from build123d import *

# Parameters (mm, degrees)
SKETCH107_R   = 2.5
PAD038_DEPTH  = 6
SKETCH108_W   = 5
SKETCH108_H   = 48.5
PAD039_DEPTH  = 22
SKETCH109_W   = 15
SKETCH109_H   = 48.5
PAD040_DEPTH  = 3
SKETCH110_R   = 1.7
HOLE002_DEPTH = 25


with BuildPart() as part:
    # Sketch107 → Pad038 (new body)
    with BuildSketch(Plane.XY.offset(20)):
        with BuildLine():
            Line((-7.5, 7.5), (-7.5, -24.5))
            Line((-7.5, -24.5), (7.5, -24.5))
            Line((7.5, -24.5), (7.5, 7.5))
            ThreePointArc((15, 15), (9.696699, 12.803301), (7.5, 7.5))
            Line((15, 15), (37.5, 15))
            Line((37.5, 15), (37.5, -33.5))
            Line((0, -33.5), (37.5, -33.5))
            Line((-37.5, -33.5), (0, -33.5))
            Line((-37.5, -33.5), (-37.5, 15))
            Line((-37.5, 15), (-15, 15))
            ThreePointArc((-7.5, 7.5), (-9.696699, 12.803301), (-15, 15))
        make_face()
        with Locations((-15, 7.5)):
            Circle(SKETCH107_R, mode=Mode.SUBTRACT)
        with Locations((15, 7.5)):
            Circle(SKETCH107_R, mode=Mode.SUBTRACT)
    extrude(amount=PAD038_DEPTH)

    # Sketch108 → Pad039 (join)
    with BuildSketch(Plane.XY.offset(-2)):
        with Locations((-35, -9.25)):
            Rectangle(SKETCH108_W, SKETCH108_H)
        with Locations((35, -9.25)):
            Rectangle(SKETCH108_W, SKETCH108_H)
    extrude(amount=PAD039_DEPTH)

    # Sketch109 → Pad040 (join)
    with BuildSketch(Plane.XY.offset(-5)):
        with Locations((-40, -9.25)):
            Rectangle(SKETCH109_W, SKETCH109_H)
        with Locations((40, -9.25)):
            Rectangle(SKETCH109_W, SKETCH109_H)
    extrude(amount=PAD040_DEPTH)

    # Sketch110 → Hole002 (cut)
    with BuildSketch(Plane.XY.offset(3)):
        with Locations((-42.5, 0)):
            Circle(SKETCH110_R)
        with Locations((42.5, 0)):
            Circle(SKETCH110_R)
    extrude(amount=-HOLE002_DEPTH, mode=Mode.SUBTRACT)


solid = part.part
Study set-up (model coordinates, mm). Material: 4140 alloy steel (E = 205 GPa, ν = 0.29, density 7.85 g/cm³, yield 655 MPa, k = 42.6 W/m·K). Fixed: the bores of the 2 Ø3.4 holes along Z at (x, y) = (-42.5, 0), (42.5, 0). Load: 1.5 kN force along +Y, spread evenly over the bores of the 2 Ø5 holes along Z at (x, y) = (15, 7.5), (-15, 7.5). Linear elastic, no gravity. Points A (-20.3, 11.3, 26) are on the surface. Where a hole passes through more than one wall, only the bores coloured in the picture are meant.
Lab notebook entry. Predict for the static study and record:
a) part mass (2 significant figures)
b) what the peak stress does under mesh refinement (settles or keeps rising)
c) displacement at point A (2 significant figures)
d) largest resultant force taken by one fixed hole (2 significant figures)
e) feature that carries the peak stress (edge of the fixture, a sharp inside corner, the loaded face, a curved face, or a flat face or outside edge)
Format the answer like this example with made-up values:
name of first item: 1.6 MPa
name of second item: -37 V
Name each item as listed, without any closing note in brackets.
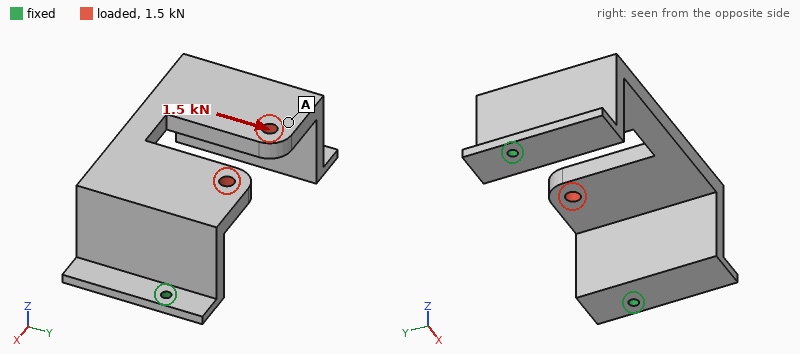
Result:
part mass: 260 g
what the peak stress does under mesh refinement: keeps rising
displacement at point A: 0.23 mm
largest resultant force taken by one fixed hole: 760 N
feature that carries the peak stress: edge of the fixture
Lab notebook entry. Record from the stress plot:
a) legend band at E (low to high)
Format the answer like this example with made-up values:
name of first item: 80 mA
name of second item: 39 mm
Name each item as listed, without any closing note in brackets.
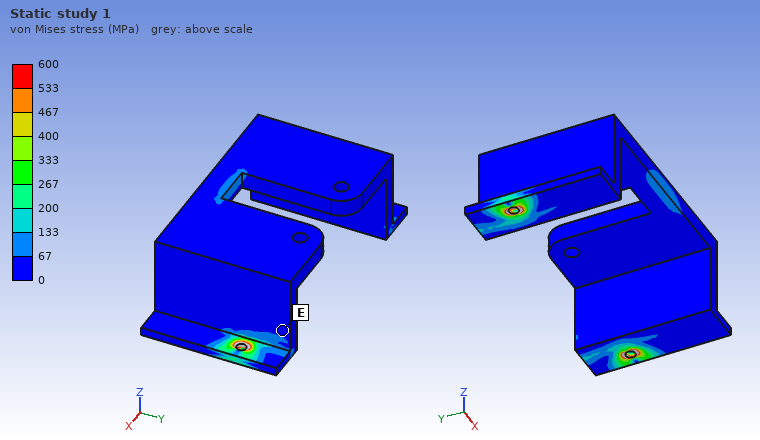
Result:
legend band at E: 0 to 67 MPa
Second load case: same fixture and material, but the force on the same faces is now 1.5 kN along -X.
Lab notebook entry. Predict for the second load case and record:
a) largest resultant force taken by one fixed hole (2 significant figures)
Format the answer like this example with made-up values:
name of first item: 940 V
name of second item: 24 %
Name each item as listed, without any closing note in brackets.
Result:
largest resultant force taken by one fixed hole: 830 N
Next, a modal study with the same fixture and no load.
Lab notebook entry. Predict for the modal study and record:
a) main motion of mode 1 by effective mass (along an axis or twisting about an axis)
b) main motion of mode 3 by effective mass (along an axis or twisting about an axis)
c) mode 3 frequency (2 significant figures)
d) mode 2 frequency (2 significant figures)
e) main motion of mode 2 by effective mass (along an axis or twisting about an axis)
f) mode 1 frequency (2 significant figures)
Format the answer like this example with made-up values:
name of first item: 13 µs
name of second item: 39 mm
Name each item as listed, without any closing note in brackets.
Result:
main motion of mode 1 by effective mass: along Y
main motion of mode 3 by effective mass: along X
mode 3 frequency: 2000 Hz
mode 2 frequency: 1500 Hz
main motion of mode 2 by effective mass: along X
mode 1 frequency: 860 Hz
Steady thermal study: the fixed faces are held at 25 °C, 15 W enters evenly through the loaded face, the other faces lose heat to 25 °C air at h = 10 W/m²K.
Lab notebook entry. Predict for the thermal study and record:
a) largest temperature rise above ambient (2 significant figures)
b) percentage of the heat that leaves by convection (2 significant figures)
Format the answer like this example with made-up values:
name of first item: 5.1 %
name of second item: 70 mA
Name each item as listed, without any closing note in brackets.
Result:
largest temperature rise above ambient: 57 K
percentage of the heat that leaves by convection: 29 %
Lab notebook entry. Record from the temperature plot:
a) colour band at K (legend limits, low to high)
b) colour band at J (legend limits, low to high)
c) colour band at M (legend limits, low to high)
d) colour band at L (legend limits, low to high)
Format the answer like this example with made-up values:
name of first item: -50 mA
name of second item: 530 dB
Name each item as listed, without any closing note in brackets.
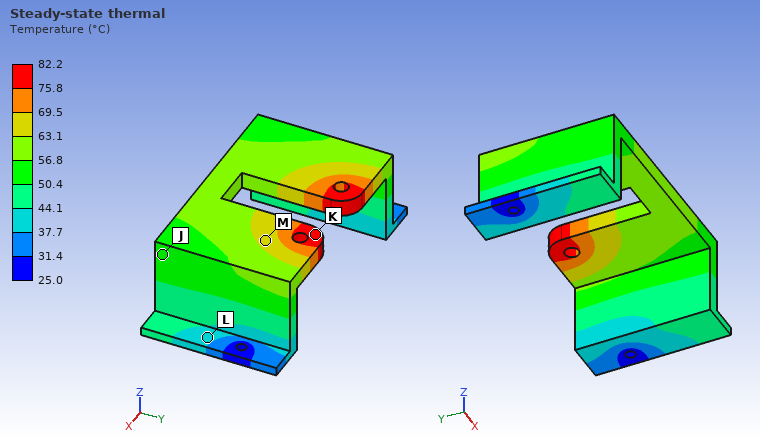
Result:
colour band at K: 75.8 to 82.2 °C
colour band at J: 50.4 to 56.8 °C
colour band at M: 63.1 to 69.5 °C
colour band at L: 37.7 to 44.1 °C
